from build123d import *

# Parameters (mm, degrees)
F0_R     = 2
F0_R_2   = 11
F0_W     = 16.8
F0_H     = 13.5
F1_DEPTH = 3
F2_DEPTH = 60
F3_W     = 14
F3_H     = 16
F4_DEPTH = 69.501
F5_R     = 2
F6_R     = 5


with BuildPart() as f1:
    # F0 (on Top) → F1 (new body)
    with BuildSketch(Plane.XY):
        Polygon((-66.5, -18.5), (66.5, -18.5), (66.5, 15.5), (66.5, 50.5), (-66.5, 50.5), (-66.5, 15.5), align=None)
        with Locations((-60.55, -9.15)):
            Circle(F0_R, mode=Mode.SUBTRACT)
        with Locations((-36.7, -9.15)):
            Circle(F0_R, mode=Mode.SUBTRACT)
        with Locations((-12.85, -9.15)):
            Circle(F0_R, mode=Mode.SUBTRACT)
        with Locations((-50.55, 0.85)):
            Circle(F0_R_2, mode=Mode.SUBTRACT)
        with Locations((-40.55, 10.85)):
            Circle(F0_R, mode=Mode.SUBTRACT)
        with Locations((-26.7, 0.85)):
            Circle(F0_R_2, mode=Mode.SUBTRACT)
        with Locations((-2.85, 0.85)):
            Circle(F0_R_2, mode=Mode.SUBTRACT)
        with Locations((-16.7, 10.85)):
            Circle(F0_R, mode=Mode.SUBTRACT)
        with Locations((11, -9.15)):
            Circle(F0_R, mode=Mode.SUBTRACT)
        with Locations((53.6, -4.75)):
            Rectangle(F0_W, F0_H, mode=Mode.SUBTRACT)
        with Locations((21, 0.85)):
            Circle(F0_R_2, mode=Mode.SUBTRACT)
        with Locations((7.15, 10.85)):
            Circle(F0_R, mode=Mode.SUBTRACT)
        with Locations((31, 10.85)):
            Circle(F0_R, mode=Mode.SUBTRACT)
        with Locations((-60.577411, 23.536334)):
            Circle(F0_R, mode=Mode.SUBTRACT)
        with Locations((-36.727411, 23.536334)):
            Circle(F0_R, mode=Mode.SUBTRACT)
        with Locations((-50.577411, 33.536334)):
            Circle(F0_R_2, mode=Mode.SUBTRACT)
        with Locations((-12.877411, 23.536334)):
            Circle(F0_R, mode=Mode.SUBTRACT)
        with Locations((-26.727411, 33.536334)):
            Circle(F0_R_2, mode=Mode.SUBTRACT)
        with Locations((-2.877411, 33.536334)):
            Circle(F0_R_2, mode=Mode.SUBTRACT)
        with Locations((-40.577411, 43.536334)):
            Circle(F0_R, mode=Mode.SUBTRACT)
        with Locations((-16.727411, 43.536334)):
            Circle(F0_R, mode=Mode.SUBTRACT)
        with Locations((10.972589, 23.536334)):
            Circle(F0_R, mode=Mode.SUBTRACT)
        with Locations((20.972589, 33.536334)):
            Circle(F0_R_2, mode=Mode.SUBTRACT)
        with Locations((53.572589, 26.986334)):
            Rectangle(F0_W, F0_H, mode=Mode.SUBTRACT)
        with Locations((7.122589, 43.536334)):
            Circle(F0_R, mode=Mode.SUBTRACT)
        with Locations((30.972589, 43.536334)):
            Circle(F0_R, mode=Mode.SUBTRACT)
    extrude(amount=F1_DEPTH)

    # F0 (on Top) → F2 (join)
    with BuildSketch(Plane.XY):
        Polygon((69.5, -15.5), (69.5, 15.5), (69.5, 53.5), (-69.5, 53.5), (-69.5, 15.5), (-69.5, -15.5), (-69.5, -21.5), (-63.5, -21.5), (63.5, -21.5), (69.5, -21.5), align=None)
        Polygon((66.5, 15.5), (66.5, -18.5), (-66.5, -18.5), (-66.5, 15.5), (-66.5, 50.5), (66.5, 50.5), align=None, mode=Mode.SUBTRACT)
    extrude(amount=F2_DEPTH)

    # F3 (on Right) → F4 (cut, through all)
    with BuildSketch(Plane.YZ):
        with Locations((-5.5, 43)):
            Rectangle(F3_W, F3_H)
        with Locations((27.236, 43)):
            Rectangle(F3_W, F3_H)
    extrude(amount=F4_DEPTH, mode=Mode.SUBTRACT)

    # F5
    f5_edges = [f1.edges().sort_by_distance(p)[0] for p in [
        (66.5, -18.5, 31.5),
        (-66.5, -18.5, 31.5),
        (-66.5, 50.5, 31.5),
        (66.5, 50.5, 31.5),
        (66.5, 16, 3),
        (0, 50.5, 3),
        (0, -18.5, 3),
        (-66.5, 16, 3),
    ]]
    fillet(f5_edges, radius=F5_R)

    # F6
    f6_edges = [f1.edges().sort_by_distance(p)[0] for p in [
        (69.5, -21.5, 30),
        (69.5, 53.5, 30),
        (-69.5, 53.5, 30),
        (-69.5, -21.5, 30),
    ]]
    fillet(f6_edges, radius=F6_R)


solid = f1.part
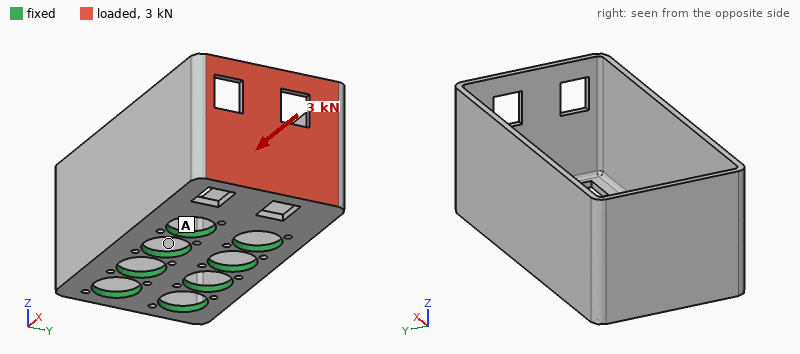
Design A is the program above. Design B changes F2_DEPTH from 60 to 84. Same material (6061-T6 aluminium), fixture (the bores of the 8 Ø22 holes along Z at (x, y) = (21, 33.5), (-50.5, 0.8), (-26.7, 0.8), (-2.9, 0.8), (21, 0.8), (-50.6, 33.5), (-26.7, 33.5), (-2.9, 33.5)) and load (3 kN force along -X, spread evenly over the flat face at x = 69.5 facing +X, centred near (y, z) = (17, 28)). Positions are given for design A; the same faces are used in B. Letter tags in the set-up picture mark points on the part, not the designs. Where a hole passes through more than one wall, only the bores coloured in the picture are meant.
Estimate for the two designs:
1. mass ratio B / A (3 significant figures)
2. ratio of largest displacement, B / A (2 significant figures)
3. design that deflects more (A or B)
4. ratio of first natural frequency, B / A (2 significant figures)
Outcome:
1.33
0.90
A
0.77
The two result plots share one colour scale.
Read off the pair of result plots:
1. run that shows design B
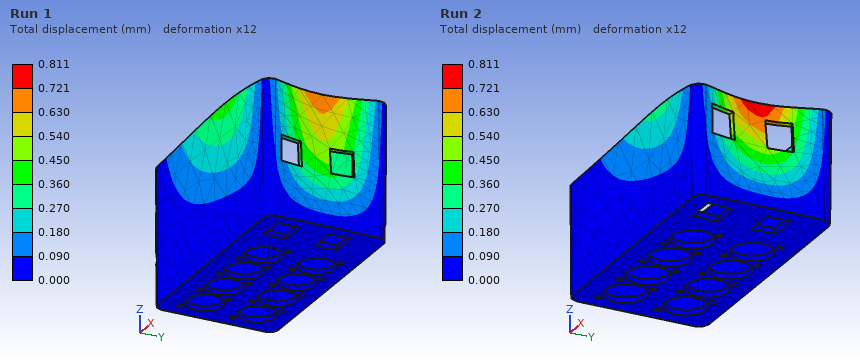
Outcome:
Run 1
